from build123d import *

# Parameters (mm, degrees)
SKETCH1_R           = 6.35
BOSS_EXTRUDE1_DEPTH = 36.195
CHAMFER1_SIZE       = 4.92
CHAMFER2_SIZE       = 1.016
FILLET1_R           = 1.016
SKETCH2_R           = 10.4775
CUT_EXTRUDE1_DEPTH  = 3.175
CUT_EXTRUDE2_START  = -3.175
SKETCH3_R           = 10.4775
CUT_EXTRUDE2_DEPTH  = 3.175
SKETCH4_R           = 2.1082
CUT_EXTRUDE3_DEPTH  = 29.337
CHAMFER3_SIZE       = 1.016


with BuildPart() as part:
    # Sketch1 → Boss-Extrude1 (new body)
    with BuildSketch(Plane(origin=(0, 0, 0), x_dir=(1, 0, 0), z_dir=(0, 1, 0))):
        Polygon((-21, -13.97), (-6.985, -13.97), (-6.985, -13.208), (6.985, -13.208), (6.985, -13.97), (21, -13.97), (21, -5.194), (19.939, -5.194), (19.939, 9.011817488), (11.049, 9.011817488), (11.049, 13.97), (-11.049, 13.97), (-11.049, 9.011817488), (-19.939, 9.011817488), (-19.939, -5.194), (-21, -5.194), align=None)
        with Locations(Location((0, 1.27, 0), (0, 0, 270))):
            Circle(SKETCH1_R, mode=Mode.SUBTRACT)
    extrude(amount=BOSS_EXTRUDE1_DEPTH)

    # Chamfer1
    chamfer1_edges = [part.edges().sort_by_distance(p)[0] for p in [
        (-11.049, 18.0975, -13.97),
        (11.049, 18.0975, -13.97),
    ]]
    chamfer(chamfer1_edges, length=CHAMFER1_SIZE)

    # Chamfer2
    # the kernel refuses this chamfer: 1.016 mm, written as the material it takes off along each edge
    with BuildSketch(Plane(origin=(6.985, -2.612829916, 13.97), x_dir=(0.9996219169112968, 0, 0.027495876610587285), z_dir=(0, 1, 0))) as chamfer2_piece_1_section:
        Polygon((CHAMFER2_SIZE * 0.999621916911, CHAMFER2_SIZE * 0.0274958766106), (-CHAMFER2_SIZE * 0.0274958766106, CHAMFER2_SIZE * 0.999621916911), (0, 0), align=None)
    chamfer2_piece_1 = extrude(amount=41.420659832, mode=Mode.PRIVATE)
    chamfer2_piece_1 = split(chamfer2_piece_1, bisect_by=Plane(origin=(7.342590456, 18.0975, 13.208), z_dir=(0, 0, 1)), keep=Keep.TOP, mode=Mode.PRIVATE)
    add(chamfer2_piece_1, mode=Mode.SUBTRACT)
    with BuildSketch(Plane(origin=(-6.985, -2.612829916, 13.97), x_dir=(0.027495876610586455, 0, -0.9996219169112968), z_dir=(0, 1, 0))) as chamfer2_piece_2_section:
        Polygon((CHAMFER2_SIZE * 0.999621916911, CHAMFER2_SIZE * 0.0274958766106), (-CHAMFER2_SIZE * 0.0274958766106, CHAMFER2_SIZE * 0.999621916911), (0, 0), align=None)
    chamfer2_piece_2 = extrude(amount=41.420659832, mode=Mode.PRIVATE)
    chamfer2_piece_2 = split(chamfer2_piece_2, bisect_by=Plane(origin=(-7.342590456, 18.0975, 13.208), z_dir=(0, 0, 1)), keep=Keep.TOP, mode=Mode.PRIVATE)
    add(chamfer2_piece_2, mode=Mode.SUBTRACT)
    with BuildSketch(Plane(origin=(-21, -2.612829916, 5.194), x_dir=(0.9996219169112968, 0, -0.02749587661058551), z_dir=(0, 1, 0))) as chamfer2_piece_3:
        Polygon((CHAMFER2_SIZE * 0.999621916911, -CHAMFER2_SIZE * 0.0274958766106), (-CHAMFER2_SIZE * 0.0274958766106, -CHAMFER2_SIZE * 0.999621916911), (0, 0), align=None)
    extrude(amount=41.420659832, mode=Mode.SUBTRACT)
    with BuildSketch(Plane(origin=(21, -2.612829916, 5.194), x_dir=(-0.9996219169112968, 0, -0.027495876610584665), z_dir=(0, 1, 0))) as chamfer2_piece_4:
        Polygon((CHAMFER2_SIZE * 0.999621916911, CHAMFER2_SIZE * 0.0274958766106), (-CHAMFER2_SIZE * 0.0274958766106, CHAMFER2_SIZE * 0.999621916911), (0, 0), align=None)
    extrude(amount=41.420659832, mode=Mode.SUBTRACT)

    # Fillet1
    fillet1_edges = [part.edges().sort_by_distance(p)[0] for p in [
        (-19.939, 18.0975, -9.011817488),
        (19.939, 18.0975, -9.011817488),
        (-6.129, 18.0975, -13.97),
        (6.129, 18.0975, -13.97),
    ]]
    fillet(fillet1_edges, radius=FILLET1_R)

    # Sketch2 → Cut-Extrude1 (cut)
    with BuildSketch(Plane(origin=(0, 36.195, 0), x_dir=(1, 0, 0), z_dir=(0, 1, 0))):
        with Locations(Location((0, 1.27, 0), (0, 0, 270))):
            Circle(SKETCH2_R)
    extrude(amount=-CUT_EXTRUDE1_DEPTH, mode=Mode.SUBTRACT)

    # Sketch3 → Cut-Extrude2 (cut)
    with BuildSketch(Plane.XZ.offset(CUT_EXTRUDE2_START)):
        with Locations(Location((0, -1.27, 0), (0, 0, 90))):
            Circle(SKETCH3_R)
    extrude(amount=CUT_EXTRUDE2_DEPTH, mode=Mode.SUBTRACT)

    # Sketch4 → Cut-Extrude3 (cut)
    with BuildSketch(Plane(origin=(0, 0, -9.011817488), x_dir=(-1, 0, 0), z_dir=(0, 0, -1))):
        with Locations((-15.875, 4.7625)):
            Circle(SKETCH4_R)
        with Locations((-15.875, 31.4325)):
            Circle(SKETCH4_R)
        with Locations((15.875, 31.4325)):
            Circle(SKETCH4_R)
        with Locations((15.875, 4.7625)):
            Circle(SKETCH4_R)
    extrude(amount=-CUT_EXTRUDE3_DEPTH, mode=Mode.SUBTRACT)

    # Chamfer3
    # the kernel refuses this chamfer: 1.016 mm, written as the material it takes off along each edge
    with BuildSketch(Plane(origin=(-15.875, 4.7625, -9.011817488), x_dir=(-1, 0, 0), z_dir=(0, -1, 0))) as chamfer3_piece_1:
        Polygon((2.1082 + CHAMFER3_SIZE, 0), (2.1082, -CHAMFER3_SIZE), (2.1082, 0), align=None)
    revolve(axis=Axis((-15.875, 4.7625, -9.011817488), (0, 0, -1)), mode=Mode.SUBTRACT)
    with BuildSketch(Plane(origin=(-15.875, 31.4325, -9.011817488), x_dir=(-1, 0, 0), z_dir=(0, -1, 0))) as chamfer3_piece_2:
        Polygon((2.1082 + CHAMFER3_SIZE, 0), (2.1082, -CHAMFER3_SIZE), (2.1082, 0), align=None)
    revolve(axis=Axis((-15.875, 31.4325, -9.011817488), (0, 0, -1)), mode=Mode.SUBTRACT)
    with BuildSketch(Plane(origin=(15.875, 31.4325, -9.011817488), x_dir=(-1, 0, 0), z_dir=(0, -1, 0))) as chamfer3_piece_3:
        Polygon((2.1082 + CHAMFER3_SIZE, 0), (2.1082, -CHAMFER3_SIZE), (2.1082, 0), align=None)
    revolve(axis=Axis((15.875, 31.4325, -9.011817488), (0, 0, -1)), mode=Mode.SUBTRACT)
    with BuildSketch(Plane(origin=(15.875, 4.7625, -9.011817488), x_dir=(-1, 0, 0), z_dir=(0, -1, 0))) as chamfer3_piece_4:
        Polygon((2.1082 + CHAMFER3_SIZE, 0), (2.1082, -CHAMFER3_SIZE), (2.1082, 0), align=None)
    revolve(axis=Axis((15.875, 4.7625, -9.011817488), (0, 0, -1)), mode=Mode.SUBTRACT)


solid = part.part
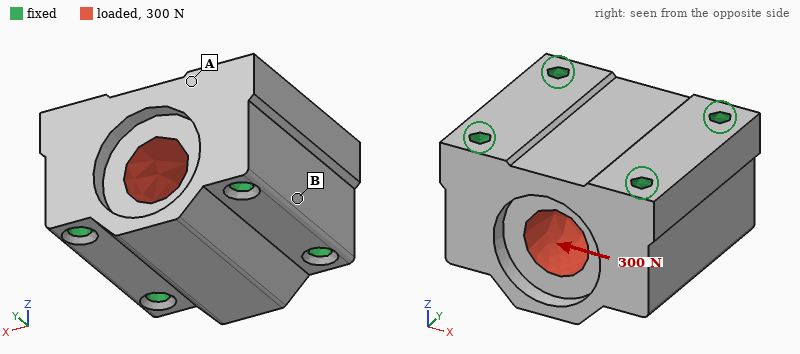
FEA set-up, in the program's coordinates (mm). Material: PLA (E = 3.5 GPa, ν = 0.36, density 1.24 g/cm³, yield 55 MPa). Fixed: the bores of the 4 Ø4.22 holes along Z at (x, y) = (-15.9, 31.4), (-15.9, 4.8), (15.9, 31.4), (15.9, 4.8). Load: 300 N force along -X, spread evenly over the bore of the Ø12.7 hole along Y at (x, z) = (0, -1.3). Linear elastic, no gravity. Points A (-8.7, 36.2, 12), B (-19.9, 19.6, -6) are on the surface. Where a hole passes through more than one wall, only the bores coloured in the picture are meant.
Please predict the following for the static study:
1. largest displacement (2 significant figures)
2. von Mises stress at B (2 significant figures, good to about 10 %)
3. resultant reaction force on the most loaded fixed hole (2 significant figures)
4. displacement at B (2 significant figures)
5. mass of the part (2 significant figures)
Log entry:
2.3 µm
0.22 MPa
80 N
1.5 µm
36 g
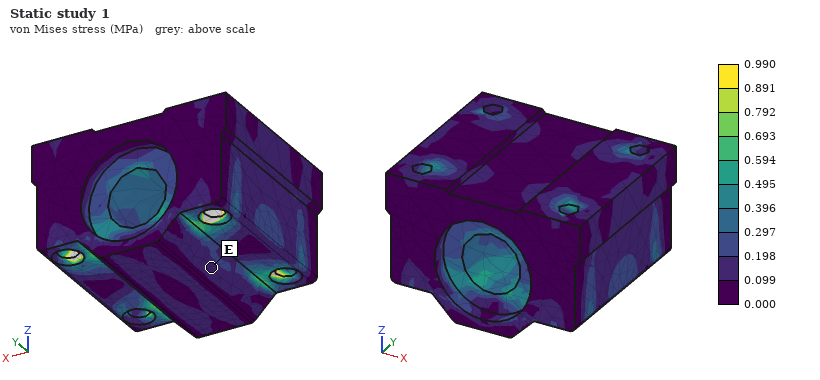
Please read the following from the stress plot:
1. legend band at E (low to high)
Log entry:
0.099 to 0.198 MPa
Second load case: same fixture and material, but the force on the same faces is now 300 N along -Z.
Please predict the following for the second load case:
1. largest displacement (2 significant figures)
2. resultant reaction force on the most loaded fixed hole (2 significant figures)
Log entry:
3.6 µm
76 N
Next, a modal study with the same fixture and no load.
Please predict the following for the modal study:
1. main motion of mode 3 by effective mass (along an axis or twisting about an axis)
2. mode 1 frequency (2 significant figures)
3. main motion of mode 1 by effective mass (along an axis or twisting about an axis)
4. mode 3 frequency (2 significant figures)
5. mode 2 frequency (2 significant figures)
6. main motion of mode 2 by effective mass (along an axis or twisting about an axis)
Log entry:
along X
13 kHz
along Z
15 kHz
14 kHz
along Y
